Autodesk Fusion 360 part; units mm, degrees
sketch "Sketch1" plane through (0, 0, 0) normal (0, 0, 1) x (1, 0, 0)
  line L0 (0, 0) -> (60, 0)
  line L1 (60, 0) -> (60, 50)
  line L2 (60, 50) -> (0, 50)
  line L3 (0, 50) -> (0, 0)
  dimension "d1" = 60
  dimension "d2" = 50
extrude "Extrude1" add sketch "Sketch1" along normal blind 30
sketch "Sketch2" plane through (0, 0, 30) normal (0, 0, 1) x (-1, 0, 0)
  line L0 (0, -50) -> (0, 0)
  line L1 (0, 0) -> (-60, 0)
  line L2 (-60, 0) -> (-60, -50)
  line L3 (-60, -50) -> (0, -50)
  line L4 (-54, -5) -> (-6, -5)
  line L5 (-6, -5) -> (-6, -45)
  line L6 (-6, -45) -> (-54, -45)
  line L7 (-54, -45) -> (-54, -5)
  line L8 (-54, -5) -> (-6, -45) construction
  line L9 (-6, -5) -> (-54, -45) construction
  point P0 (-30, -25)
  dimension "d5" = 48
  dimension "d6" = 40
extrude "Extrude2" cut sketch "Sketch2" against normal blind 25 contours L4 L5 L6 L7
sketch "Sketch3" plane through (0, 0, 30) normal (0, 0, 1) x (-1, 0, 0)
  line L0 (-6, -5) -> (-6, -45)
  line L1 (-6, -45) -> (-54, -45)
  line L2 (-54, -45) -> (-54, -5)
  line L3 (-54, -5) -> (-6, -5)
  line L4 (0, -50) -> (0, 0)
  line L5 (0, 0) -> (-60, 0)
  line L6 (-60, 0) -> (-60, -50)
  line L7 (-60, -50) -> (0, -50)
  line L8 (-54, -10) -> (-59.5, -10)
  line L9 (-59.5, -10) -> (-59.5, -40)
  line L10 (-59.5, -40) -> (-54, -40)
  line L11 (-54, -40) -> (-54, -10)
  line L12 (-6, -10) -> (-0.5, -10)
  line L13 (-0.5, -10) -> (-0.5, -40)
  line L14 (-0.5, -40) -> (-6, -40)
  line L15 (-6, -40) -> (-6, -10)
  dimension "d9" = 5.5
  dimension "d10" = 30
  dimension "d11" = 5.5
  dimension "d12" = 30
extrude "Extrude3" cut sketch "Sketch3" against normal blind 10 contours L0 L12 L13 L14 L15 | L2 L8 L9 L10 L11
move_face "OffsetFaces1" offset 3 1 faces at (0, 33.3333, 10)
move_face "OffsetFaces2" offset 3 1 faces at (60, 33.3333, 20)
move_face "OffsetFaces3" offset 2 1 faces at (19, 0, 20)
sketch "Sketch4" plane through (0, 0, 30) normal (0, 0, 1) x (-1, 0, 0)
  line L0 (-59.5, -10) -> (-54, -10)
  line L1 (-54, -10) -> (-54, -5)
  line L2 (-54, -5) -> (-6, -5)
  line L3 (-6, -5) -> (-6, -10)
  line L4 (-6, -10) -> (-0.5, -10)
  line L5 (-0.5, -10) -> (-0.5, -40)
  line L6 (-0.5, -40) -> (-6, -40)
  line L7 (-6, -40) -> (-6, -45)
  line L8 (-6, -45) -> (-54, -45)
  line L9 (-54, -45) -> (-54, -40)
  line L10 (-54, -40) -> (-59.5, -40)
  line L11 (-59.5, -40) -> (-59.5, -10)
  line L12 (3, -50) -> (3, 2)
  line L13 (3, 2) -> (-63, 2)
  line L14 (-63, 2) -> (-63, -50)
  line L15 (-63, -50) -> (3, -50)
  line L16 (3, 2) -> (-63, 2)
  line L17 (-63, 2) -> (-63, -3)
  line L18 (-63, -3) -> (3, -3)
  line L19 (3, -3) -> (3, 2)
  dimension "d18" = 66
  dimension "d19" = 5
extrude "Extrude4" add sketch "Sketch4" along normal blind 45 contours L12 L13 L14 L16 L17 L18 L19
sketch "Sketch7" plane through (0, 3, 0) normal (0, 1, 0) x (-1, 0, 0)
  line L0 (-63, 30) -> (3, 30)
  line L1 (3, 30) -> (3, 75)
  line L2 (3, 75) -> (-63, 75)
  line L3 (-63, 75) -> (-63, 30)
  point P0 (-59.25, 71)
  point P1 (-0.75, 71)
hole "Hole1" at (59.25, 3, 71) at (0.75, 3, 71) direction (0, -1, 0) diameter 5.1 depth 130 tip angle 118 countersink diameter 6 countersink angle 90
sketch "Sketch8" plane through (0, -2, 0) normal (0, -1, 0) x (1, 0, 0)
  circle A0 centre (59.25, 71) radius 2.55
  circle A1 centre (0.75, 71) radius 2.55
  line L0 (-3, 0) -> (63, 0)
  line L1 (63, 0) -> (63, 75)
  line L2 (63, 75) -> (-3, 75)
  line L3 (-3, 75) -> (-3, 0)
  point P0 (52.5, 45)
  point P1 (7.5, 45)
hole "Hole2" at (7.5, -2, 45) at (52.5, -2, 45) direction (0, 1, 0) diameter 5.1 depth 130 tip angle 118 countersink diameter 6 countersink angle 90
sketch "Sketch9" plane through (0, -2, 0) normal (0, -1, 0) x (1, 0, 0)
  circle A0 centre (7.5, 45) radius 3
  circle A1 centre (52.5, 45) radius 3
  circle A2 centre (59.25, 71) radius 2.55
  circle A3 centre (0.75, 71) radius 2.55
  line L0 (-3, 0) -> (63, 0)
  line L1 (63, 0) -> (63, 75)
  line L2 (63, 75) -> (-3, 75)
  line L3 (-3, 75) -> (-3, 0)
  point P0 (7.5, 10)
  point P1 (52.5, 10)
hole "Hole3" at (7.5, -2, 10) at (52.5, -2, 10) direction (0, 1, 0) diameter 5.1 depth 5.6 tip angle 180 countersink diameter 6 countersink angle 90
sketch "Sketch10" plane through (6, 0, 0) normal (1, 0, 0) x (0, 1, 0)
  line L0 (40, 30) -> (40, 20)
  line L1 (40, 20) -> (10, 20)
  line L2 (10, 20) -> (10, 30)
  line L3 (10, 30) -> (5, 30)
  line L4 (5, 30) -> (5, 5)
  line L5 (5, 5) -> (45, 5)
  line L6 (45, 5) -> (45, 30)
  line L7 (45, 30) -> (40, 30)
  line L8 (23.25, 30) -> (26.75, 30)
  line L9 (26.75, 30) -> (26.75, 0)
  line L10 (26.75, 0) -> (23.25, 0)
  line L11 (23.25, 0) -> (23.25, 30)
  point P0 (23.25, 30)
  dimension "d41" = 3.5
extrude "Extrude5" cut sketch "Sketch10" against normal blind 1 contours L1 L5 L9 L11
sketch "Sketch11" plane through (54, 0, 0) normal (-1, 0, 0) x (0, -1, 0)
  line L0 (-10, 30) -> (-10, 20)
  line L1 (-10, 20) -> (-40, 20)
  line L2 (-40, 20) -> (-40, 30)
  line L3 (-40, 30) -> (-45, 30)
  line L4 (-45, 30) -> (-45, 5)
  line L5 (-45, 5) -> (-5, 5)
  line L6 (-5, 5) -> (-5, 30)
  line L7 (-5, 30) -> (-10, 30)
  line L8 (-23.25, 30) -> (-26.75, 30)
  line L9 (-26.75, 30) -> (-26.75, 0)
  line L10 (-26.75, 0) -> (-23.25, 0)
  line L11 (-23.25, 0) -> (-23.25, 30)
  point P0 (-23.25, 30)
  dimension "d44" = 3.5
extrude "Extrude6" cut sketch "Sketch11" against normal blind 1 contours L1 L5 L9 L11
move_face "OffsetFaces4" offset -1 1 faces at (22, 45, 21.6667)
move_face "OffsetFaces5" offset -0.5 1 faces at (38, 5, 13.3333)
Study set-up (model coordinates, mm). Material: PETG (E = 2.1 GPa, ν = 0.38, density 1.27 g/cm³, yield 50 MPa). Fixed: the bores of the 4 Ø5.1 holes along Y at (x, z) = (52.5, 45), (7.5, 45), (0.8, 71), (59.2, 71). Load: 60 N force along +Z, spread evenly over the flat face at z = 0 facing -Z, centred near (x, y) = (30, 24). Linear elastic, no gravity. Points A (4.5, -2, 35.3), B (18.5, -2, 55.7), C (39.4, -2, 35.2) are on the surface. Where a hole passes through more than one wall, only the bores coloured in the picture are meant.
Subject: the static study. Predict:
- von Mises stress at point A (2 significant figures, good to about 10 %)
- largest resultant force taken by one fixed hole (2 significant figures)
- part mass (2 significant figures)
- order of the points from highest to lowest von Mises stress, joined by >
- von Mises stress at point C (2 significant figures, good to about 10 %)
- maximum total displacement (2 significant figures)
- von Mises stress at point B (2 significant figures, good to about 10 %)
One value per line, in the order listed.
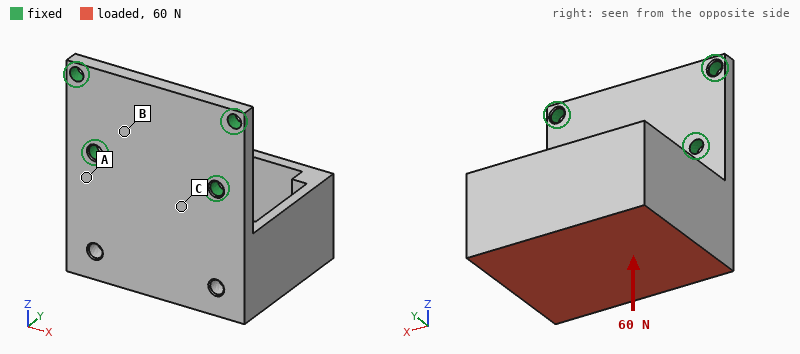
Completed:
5.2 MPa
28 N
81 g
A > C > B
3.7 MPa
1.2 mm
0.79 MPa
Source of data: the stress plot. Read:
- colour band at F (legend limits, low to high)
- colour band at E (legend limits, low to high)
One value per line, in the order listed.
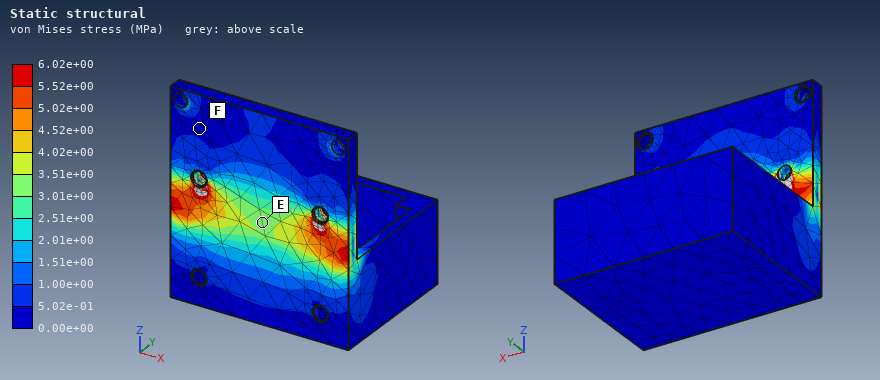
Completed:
0.00e+00 to 5.02e-01 MPa
3.01e+00 to 3.51e+00 MPa
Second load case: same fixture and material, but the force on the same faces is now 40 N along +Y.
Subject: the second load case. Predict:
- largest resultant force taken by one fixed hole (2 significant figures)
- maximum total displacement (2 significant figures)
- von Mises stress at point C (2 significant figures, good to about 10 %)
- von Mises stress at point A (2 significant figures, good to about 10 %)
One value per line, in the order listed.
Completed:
30 N
1.2 mm
3.8 MPa
5.3 MPa
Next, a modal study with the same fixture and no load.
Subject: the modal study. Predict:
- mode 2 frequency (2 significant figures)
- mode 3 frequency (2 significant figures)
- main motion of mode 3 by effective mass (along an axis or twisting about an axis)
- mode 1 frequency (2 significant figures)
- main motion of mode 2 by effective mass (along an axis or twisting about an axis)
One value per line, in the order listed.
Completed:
320 Hz
840 Hz
along Y
140 Hz
along X
